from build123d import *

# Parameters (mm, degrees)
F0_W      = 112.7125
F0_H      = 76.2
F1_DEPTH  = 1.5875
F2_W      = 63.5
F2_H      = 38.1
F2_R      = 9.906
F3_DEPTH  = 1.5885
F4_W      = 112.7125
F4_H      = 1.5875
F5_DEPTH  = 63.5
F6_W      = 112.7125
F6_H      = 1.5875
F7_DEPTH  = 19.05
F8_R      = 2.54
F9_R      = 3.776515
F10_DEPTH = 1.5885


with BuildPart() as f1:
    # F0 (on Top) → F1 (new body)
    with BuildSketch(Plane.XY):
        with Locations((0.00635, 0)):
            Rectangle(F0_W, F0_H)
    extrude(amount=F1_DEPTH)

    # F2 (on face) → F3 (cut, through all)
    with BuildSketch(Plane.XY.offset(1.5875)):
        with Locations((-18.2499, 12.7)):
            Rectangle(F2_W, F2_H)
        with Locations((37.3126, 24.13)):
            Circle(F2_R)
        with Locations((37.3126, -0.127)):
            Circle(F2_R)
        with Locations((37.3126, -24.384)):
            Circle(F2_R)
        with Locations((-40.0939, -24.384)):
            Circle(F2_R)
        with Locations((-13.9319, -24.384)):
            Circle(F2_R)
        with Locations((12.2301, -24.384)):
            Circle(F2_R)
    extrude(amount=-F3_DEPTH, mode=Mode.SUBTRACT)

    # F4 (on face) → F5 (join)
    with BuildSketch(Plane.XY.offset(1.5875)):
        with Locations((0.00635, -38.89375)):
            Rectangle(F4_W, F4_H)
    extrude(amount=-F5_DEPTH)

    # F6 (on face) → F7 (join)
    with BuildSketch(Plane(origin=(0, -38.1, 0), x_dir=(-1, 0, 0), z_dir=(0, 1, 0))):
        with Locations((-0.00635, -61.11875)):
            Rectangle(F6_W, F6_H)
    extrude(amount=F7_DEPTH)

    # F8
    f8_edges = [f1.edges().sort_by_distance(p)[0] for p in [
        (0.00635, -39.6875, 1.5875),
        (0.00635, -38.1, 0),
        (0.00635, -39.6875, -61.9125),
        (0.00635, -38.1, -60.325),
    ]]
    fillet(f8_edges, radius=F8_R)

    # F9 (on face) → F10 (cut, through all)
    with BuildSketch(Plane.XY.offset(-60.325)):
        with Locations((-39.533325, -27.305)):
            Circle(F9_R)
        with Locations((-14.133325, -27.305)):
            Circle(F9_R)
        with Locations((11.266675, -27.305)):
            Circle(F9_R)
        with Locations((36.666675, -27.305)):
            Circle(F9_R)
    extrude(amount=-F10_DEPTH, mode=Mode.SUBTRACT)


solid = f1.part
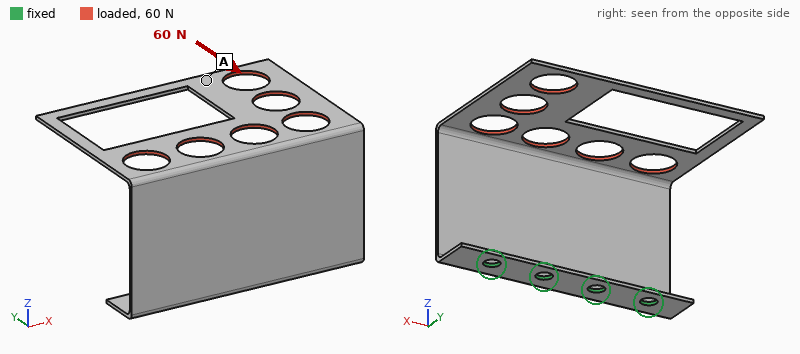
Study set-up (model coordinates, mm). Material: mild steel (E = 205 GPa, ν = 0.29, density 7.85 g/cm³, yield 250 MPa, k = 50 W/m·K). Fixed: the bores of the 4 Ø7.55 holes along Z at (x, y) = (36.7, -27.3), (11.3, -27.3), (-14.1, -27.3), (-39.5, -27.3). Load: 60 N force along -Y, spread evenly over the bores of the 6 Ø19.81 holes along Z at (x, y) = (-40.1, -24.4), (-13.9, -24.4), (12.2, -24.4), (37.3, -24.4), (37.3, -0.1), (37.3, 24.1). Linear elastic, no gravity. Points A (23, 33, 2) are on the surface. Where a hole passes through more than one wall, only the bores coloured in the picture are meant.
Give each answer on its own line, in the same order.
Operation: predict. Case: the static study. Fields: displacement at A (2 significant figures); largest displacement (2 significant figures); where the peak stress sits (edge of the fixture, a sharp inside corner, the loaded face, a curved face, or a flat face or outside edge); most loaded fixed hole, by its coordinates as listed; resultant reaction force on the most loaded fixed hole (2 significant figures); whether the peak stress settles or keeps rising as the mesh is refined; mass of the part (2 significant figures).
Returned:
1.5 mm
1.6 mm
edge of the fixture
(36.7, -27.3)
25 N
keeps rising
170 g
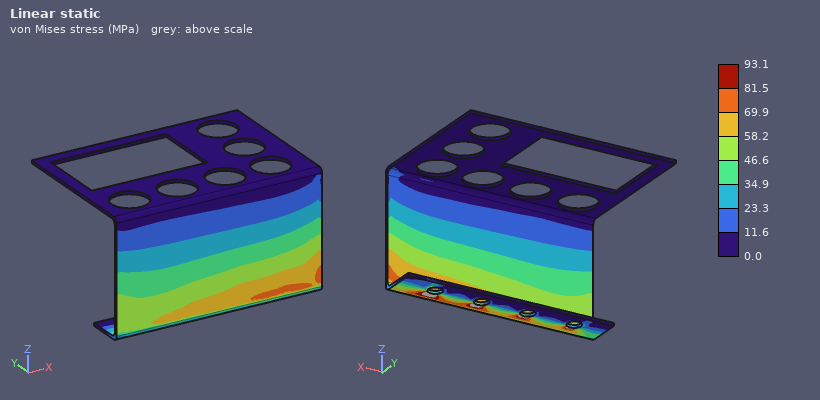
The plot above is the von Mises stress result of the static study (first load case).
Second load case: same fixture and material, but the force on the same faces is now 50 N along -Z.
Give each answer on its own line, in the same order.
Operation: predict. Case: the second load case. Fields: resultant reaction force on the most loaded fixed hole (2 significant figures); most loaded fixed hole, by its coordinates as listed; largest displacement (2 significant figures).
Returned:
20 N
(36.7, -27.3)
1.6 mm
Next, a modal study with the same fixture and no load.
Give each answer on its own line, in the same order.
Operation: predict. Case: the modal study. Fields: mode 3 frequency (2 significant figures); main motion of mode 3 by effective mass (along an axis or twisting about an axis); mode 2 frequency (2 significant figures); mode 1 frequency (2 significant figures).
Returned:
240 Hz
along Y
200 Hz
110 Hz
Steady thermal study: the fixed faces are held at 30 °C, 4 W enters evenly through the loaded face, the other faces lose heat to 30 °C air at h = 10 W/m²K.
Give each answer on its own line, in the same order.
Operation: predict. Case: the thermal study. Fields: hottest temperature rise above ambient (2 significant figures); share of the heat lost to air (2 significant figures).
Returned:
28 K
68 %
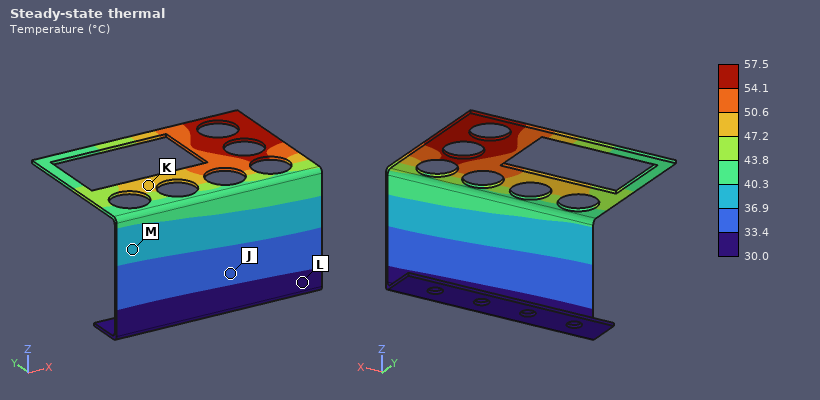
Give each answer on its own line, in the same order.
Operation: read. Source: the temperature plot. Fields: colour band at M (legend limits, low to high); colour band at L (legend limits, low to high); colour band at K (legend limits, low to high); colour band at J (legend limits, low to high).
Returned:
36.9 to 40.3 °C
30.0 to 33.4 °C
47.2 to 50.6 °C
33.4 to 36.9 °C
